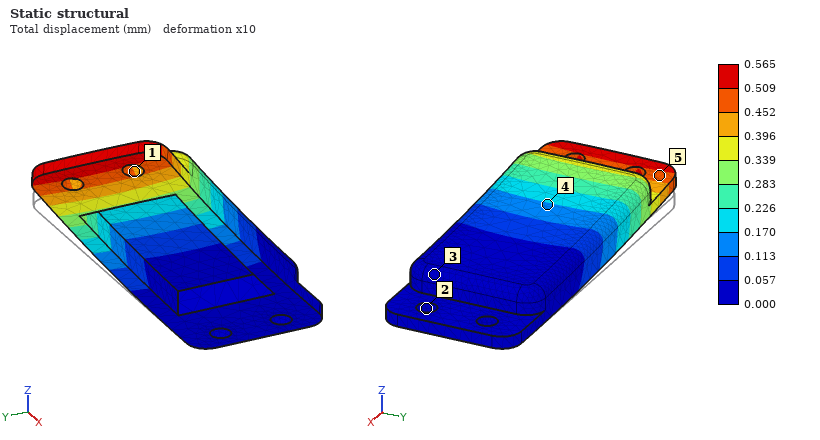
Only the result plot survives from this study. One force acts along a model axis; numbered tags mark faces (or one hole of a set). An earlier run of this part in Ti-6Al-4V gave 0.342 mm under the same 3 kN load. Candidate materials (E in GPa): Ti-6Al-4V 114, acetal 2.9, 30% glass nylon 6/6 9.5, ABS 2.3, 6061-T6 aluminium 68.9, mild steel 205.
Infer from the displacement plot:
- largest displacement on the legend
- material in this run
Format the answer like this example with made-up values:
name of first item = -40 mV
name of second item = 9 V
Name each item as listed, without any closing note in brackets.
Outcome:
largest displacement on the legend = 0.565 mm
material in this run = 6061-T6 aluminium
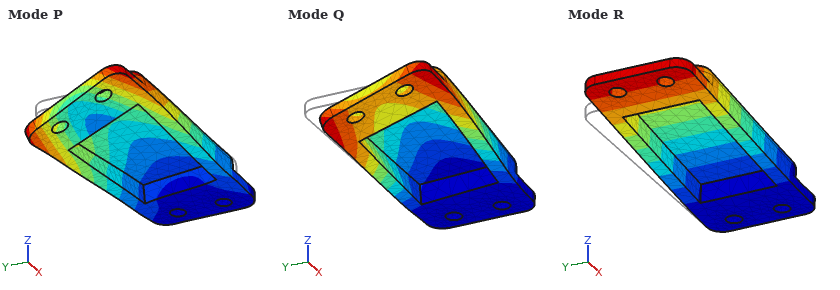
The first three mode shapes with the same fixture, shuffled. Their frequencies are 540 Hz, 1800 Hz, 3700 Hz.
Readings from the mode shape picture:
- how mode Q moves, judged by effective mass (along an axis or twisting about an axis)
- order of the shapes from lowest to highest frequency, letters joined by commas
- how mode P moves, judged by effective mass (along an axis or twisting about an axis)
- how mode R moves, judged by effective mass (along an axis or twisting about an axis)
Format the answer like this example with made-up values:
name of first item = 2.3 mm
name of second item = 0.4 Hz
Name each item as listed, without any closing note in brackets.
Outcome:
how mode Q moves, judged by effective mass = along Y
order of the shapes from lowest to highest frequency, letters joined by commas = R, Q, P
how mode P moves, judged by effective mass = along Y
how mode R moves, judged by effective mass = along Z
